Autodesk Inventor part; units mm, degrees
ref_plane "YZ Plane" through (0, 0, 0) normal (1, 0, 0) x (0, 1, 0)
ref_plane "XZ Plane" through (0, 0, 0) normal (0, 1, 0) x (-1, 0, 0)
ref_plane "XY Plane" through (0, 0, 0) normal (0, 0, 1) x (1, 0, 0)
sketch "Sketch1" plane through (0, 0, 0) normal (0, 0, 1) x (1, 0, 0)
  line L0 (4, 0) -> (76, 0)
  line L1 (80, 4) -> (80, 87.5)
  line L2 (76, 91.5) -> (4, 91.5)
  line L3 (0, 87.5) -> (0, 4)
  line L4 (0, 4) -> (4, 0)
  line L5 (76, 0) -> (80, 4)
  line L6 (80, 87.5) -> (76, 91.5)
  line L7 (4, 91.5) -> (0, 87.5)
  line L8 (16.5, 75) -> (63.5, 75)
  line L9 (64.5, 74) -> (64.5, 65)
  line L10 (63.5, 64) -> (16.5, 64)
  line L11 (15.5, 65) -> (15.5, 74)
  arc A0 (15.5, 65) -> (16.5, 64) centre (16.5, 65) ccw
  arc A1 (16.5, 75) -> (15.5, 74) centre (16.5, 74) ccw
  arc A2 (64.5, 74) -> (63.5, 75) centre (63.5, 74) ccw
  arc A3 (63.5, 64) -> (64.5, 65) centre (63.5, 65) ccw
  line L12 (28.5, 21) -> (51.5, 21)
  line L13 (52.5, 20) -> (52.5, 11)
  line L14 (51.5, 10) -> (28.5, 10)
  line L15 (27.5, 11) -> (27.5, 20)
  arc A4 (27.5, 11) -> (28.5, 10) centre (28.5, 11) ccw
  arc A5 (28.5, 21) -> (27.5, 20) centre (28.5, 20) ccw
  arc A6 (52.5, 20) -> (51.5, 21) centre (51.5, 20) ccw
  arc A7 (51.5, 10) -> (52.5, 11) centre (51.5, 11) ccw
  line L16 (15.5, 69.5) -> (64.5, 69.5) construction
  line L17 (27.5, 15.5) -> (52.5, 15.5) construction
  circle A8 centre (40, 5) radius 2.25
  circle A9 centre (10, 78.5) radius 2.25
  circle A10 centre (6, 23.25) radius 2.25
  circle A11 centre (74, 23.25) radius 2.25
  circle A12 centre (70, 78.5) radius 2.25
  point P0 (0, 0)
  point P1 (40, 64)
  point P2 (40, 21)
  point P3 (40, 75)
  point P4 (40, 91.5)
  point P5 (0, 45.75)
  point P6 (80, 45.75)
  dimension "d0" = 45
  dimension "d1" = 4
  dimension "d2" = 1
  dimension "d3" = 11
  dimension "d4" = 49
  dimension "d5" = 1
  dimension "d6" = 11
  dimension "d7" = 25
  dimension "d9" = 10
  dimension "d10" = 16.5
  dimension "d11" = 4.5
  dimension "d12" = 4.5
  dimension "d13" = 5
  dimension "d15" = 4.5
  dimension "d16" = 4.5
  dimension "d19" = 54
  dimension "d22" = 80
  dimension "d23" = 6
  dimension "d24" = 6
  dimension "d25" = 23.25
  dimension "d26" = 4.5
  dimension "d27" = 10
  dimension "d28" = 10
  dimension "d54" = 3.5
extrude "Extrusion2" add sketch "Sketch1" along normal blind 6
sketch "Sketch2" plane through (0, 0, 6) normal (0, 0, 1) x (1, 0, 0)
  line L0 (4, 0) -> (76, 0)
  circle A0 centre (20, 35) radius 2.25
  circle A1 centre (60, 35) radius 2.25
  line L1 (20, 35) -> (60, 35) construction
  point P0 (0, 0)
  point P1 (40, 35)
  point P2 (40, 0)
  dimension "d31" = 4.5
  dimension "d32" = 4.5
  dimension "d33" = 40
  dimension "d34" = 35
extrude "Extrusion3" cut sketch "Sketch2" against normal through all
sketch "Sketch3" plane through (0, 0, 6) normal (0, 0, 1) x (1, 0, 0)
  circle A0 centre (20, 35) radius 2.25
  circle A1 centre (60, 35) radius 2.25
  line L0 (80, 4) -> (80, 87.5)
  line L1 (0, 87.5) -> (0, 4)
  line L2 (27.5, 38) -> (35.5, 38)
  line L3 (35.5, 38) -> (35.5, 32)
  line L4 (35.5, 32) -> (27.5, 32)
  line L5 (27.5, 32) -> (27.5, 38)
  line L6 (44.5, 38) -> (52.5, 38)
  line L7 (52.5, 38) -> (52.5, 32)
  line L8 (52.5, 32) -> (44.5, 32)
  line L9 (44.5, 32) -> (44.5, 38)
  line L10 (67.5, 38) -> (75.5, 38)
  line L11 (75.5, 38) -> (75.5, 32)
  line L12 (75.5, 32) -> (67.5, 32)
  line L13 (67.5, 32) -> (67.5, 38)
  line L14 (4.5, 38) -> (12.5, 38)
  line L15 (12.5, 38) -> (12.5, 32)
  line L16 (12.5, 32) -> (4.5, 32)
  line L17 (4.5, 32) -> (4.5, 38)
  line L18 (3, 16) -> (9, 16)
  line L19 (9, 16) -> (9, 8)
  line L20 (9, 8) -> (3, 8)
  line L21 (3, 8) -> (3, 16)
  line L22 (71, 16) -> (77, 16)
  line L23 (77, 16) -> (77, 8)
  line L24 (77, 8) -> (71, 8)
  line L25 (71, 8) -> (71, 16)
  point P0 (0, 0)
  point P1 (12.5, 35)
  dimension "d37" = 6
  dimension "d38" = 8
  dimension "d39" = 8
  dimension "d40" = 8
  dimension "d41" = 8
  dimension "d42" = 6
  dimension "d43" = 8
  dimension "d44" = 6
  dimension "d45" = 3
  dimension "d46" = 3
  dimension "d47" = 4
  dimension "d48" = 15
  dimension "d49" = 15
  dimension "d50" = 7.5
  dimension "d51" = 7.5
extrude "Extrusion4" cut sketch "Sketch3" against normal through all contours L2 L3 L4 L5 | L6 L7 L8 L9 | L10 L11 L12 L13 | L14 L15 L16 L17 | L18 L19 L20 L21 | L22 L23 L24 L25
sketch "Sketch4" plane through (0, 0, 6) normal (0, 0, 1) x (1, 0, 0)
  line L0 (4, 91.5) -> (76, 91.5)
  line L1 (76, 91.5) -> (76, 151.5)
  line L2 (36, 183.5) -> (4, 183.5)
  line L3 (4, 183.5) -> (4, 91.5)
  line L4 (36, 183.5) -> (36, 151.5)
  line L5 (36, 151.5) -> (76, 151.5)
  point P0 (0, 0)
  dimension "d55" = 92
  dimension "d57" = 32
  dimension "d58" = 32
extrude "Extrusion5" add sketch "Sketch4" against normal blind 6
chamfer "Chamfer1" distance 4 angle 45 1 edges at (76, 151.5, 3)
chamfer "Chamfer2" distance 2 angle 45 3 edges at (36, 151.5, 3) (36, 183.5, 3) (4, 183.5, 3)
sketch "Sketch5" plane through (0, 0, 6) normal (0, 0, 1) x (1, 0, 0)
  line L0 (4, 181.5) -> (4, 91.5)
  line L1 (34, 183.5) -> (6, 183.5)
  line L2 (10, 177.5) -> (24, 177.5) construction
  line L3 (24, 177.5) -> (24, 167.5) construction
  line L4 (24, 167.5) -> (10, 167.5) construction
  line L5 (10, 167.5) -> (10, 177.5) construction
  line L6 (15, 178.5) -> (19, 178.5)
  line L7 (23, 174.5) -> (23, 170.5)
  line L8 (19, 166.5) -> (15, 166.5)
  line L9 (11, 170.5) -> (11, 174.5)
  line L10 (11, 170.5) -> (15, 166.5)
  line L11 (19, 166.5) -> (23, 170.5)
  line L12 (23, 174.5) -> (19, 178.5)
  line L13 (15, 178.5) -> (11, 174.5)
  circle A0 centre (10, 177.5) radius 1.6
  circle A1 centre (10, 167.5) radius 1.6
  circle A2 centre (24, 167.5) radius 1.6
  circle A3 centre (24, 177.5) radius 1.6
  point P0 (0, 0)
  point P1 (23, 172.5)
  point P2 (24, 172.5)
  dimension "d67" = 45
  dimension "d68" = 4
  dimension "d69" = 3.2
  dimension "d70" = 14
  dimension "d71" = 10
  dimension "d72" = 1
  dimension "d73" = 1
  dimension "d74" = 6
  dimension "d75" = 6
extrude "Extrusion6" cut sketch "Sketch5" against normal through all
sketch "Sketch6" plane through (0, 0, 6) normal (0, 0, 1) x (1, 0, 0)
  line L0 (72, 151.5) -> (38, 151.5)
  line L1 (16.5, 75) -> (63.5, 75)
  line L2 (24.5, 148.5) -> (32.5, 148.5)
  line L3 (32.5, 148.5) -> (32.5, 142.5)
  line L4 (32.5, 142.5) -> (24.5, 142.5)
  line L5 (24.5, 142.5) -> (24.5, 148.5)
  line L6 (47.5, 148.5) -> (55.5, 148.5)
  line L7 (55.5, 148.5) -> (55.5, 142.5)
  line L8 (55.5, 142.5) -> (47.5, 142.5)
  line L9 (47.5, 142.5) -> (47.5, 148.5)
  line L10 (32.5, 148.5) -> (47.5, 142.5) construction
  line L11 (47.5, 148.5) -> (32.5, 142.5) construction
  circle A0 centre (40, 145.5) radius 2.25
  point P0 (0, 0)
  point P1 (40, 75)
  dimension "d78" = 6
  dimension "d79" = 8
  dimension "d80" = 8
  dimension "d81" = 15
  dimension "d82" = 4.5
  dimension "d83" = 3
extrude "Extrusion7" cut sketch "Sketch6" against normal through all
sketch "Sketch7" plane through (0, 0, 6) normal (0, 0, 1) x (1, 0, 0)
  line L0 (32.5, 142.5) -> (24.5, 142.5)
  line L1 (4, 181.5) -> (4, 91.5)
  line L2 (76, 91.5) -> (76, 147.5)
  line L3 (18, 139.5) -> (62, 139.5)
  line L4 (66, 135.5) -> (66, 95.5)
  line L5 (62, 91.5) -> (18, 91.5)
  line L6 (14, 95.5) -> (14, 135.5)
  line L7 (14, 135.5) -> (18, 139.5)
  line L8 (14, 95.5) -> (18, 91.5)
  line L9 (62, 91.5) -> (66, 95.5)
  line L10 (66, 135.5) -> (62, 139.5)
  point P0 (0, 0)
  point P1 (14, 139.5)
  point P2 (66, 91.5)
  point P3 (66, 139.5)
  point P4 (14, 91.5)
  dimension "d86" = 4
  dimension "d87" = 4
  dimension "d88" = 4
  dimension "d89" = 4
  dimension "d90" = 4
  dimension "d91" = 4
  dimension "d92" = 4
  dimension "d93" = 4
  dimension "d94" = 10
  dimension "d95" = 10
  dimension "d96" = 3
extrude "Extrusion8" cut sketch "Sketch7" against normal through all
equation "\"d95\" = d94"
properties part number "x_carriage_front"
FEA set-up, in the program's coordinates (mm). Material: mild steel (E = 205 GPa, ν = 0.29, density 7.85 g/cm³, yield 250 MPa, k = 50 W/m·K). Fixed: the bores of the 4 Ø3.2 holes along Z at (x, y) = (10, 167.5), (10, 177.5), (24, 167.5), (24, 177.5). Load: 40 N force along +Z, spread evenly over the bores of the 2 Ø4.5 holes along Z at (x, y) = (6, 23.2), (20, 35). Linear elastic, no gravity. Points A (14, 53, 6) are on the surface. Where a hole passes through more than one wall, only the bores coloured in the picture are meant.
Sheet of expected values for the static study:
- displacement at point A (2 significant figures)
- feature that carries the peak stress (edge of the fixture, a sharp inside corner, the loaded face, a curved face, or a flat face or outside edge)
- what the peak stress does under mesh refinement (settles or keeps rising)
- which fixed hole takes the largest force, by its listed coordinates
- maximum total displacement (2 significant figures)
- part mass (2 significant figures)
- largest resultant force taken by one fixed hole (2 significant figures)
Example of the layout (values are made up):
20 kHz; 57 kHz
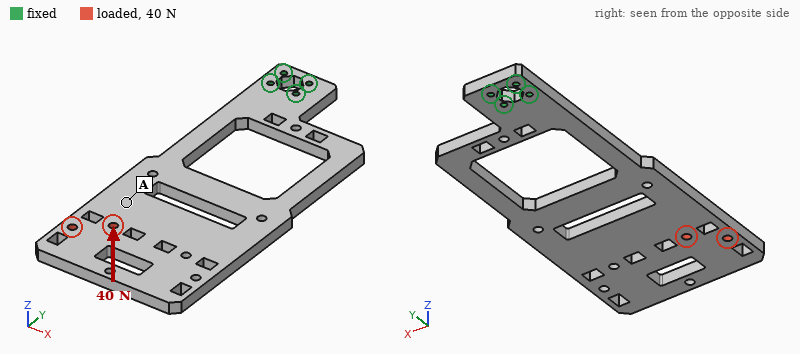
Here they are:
0.35 mm; edge of the fixture; keeps rising; (24, 167.5); 0.60 mm; 410 g; 110 N
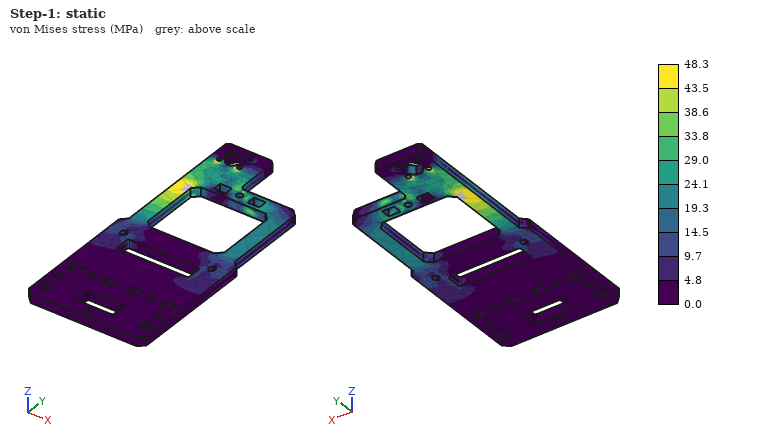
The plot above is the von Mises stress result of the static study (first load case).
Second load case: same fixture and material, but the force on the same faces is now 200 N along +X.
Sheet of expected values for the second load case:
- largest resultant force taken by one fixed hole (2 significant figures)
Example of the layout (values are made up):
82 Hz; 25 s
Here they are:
1.3 kN
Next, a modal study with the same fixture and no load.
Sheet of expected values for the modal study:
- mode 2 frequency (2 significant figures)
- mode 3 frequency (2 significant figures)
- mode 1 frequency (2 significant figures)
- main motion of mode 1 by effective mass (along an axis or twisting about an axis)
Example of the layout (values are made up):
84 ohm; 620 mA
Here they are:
400 Hz; 420 Hz; 97 Hz; along Z
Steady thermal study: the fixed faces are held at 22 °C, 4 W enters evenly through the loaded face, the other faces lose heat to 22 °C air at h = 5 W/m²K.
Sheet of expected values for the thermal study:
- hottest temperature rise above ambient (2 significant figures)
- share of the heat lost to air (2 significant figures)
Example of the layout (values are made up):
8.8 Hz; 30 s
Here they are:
38 K; 65 %
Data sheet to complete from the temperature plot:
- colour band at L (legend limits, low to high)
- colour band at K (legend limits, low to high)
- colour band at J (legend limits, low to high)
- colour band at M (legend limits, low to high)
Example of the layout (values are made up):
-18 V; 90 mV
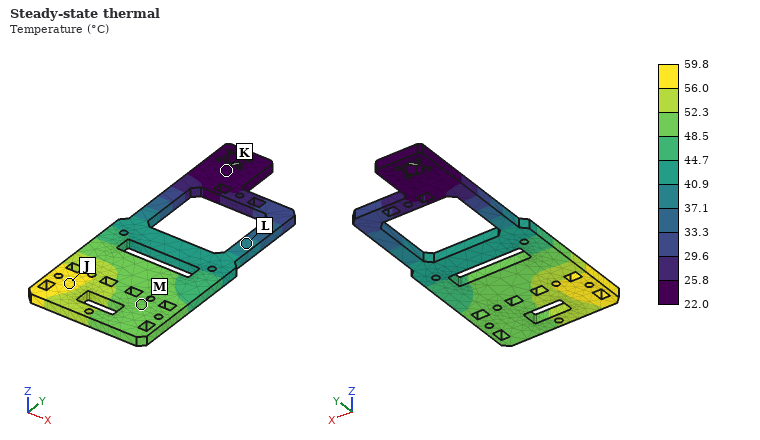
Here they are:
37.1 to 40.9 °C; 22.0 to 25.8 °C; 56.0 to 59.8 °C; 48.5 to 52.3 °C
